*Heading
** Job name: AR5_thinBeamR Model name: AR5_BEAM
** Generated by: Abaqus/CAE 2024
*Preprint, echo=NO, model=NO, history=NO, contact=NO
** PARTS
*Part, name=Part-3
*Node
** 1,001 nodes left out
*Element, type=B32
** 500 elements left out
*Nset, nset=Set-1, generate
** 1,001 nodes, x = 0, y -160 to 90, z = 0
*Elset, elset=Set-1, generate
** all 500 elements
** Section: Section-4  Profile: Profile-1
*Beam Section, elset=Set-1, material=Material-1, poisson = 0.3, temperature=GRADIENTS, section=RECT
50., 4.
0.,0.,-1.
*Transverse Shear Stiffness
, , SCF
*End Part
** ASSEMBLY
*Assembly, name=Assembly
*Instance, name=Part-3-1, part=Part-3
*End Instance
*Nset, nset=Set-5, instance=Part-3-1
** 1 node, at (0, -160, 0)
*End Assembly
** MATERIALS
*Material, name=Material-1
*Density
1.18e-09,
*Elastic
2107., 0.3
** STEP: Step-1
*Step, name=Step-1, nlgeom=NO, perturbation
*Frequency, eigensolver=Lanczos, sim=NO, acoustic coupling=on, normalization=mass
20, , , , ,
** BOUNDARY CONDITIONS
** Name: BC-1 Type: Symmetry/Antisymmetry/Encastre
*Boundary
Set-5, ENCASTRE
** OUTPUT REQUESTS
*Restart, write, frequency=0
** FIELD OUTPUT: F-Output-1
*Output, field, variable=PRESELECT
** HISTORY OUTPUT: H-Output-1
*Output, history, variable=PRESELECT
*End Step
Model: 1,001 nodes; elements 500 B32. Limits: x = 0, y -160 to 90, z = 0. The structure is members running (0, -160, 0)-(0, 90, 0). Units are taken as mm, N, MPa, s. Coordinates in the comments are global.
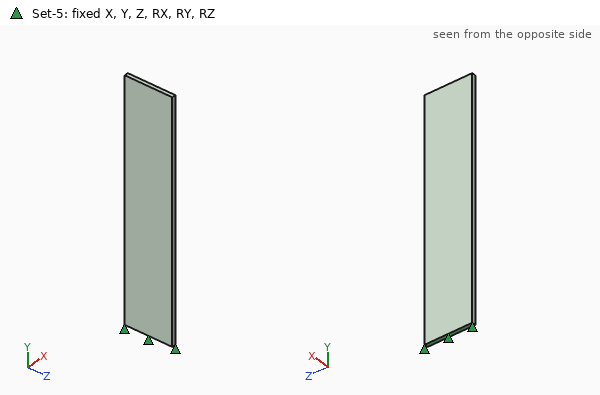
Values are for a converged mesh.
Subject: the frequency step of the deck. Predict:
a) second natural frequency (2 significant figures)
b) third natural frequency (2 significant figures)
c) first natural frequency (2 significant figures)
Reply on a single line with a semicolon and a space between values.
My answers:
88 Hz; 130 Hz; 14 Hz
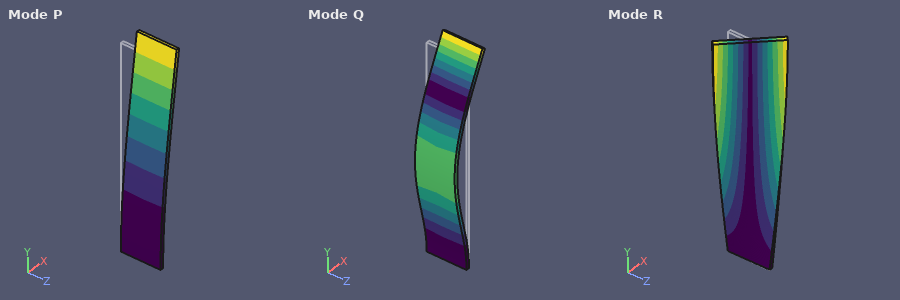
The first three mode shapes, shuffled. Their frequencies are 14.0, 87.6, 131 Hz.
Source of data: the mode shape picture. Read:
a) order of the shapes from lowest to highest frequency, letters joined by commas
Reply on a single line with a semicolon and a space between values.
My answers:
P, Q, R
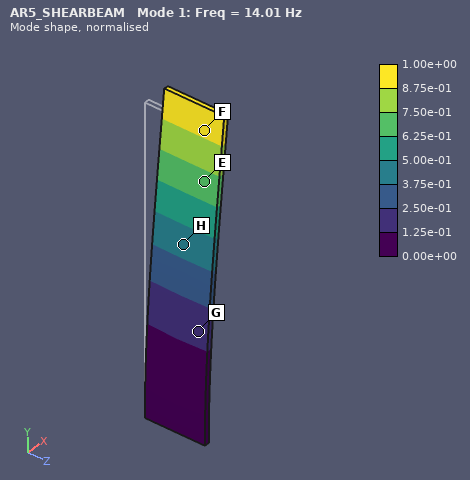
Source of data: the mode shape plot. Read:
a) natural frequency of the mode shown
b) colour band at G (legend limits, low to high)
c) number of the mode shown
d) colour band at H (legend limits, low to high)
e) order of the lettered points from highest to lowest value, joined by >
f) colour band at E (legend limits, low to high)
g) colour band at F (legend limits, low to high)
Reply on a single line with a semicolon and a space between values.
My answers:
14.01 Hz; 1.25e-01 to 2.50e-01; 1; 3.75e-01 to 5.00e-01; F > E > H > G; 6.25e-01 to 7.50e-01; 8.75e-01 to 1.00e+00
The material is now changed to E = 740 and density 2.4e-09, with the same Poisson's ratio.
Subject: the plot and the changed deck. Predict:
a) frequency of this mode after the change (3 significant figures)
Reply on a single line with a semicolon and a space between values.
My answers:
5.82 Hz
